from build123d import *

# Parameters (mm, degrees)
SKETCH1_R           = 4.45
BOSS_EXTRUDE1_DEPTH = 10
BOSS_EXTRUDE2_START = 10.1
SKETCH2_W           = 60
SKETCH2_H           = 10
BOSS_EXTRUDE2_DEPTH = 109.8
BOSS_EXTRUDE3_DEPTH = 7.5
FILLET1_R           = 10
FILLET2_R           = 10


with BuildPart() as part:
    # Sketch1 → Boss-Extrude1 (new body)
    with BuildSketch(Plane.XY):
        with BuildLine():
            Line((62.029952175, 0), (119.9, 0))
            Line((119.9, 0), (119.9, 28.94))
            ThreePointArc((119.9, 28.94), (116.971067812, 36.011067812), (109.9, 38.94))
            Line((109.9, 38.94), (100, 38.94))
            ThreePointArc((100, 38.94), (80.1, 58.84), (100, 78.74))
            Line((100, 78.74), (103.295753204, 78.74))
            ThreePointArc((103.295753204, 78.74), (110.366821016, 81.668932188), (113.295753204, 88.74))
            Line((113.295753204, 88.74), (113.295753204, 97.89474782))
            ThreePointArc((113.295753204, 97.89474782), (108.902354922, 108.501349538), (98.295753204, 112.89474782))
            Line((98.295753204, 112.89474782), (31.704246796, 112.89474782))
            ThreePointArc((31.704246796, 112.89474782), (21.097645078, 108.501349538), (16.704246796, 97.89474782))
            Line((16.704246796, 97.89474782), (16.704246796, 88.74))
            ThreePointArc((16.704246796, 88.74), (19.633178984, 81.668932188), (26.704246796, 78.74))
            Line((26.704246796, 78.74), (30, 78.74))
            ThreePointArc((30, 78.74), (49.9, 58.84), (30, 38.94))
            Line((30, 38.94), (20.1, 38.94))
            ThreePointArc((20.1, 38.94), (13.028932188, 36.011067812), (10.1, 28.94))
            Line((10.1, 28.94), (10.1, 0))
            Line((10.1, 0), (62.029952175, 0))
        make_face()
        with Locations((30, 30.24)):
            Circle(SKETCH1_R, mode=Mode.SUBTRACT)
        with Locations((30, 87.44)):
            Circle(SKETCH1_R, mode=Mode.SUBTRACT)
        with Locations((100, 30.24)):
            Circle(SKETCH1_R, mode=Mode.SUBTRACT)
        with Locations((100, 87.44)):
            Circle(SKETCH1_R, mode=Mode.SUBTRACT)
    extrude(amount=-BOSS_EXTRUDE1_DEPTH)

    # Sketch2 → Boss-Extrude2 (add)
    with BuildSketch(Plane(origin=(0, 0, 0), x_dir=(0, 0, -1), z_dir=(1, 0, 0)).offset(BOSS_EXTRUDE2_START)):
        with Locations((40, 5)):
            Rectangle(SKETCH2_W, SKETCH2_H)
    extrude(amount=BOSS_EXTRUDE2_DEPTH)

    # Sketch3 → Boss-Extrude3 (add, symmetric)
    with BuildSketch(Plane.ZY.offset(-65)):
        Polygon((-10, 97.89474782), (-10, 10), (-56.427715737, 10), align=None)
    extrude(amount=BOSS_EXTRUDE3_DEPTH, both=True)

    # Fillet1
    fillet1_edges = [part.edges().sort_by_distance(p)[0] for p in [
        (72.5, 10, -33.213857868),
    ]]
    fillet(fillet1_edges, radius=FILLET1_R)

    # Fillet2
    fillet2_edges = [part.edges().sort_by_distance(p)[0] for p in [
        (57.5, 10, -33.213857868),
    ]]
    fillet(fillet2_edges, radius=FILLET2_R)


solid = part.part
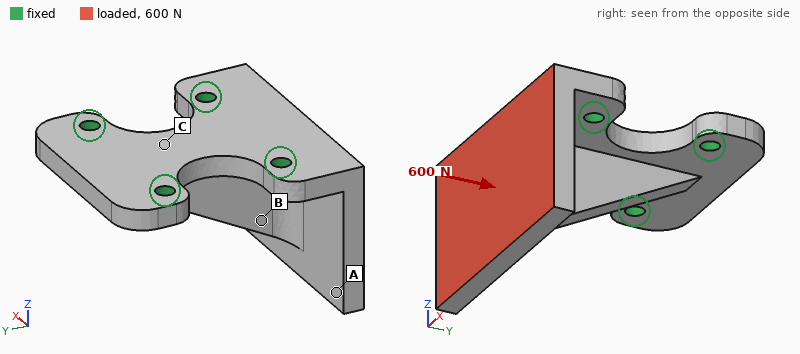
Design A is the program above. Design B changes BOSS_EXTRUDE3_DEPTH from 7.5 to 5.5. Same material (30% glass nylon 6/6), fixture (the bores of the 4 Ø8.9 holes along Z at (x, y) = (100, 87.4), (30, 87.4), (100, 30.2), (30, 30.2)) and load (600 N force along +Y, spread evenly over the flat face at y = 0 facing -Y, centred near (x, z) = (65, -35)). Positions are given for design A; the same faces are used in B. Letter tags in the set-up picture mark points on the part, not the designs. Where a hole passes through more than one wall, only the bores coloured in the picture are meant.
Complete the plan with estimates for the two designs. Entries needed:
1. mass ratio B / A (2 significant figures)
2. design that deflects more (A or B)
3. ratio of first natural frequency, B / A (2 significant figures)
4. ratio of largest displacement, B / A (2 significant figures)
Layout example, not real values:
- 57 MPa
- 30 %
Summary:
- 0.96
- B
- 0.96
- 1.1
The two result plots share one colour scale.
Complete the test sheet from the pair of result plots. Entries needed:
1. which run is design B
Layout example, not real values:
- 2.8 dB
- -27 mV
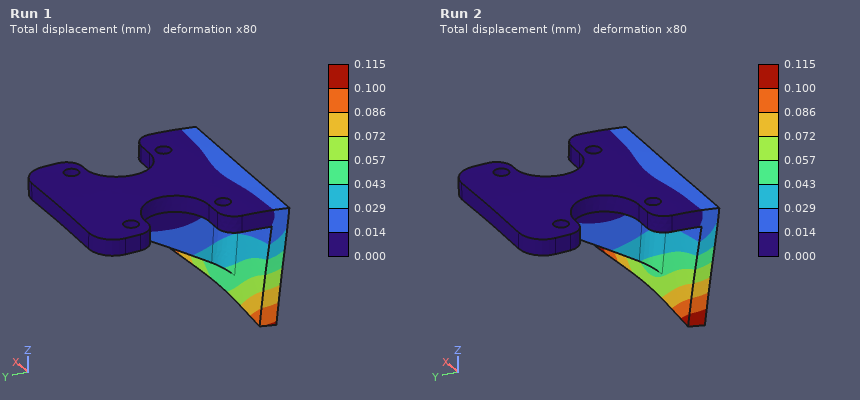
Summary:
- Run 2
